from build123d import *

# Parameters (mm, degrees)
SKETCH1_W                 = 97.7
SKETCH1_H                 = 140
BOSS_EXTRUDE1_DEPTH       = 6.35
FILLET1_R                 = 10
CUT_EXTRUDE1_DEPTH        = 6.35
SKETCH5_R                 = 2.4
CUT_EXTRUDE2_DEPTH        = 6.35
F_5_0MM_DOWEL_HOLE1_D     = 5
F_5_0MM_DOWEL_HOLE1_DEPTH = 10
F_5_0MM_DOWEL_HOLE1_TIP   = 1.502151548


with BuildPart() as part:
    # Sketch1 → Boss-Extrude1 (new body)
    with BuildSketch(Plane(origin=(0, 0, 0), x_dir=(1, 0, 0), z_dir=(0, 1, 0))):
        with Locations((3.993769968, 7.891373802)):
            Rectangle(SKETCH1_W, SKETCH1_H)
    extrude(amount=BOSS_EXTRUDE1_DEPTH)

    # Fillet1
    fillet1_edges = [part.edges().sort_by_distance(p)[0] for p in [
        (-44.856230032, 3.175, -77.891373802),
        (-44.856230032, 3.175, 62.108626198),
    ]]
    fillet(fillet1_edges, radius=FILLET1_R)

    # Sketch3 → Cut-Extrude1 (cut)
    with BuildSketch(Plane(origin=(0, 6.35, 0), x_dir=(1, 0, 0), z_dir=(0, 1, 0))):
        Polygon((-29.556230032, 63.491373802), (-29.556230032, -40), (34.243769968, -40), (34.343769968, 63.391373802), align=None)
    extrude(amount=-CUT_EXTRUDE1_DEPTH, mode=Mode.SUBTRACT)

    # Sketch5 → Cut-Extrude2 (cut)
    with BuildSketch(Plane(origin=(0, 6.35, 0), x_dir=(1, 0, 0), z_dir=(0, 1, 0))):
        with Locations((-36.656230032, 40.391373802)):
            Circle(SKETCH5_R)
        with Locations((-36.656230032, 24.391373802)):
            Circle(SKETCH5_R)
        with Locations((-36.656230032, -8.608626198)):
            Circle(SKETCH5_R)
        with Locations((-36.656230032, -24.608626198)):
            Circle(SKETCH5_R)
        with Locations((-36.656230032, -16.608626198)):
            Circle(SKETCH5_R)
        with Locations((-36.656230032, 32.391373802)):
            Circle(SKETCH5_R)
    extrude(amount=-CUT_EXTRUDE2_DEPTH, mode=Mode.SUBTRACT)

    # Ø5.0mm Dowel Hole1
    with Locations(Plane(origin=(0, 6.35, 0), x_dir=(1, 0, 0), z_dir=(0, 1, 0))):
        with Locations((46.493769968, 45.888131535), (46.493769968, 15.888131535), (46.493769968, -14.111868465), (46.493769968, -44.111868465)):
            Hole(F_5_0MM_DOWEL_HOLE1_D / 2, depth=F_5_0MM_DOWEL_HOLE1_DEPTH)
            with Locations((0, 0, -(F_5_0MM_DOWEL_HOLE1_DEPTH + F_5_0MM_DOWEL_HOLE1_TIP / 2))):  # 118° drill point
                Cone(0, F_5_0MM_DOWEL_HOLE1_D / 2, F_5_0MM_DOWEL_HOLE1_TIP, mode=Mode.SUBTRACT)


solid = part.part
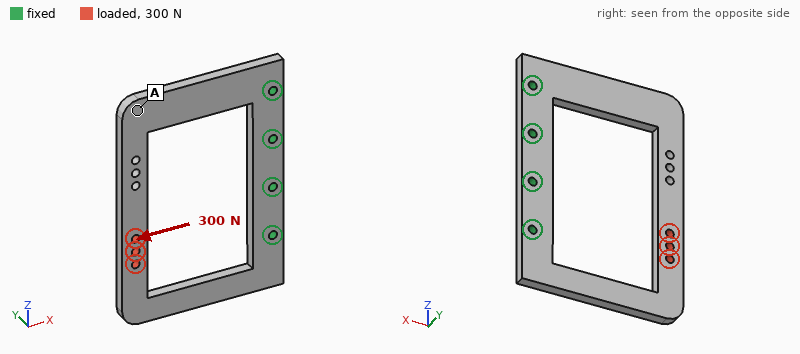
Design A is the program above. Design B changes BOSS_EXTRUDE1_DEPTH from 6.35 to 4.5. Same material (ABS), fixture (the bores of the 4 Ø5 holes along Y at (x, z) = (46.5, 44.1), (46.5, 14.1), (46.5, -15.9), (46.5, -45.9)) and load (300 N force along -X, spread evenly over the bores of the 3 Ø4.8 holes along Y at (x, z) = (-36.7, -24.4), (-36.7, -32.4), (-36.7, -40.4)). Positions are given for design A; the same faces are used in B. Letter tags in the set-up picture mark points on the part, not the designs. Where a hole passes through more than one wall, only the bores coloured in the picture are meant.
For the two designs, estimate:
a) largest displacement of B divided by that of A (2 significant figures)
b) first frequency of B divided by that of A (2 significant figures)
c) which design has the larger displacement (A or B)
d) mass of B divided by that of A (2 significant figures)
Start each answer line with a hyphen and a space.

- 1.4
- 0.72
- B
- 0.71
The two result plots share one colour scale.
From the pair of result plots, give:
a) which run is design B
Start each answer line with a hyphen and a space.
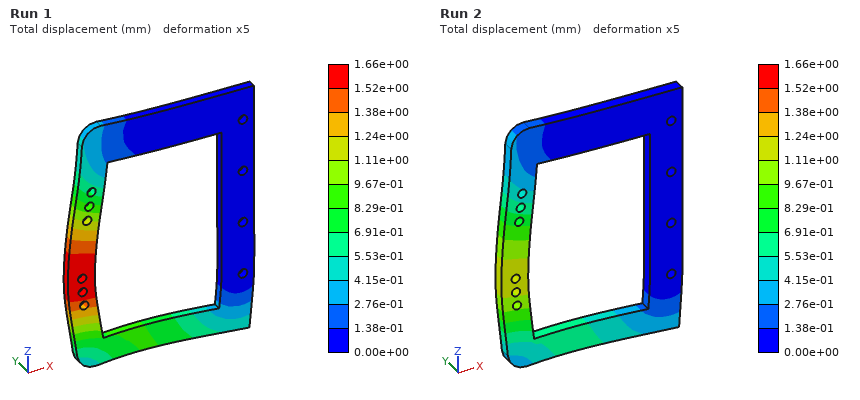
- Run 1
